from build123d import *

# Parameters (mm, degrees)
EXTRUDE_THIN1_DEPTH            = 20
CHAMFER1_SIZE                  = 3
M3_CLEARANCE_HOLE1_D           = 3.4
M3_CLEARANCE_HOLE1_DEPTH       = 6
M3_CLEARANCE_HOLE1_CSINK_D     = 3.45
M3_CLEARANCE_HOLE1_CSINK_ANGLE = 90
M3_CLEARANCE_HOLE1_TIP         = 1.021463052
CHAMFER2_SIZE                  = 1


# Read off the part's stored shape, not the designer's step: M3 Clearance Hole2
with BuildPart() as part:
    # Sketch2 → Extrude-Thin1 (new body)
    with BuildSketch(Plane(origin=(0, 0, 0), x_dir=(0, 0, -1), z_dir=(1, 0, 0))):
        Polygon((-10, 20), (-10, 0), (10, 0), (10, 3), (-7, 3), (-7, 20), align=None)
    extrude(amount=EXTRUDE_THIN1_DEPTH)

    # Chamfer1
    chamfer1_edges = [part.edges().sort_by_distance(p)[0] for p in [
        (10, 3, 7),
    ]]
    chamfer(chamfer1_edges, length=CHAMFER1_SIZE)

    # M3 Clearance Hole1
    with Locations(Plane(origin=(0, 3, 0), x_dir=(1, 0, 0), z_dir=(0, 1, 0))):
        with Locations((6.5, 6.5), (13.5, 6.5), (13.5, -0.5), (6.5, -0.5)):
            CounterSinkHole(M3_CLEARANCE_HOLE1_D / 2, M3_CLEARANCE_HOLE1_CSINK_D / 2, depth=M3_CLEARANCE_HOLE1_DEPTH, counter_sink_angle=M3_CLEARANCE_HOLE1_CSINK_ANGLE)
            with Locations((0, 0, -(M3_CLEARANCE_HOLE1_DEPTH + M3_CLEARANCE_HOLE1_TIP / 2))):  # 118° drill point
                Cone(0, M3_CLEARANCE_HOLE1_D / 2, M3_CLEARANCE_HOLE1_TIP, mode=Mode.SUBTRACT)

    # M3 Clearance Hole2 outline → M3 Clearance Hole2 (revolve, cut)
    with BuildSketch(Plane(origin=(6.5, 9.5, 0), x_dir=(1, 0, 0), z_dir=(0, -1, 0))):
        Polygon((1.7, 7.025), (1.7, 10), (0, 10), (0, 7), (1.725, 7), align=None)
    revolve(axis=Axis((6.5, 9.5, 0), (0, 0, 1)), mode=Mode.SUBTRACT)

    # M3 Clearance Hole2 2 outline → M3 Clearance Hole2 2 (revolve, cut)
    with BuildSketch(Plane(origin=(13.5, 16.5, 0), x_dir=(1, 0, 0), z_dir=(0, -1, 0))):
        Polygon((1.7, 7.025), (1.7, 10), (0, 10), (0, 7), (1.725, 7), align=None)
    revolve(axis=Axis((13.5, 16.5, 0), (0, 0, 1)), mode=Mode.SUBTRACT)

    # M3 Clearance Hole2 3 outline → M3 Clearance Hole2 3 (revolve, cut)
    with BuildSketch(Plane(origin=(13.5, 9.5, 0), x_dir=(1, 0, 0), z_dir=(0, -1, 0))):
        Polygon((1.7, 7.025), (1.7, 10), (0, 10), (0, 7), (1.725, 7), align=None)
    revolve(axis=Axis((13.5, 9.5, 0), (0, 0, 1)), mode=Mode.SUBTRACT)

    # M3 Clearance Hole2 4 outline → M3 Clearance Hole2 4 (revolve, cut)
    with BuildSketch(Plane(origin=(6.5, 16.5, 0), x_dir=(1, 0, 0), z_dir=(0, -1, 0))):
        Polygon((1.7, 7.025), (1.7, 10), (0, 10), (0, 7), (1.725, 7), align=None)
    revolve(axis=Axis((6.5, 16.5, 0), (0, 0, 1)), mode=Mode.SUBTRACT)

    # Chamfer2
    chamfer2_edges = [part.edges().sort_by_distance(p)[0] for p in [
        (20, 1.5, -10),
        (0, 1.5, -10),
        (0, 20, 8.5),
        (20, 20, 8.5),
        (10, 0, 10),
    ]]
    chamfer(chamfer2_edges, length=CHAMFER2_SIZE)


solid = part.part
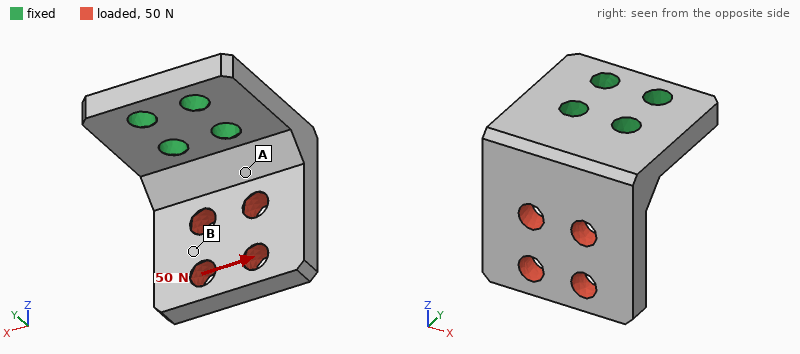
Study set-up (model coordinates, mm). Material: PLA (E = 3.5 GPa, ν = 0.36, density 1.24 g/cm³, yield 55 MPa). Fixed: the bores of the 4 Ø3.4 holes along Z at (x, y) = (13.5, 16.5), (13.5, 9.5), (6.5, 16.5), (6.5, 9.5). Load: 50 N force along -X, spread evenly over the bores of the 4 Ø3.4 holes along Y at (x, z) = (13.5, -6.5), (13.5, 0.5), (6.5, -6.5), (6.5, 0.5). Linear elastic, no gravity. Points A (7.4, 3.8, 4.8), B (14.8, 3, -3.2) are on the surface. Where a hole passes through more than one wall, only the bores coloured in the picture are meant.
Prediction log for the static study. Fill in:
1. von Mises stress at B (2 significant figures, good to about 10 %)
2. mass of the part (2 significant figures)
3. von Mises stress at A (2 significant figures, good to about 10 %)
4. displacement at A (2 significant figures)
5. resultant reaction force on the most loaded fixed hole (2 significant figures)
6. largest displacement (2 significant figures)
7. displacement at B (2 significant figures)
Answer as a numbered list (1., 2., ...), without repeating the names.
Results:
1. 2.0 MPa
2. 2.6 g
3. 7.2 MPa
4. 0.025 mm
5. 65 N
6. 0.13 mm
7. 0.081 mm
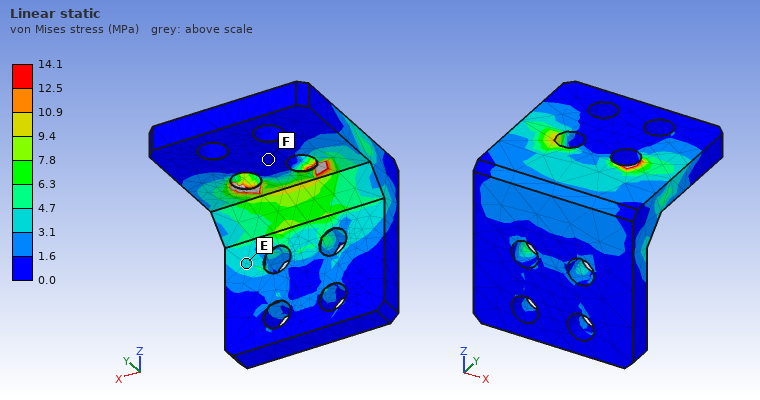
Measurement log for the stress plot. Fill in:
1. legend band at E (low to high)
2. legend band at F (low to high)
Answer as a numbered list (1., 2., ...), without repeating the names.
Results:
1. 3.1 to 4.7 MPa
2. 0.0 to 1.6 MPa
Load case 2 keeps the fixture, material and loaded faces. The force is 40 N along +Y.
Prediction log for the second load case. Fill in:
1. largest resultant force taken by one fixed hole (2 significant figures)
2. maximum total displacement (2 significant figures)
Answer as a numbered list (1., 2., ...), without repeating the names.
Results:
1. 21 N
2. 0.40 mm
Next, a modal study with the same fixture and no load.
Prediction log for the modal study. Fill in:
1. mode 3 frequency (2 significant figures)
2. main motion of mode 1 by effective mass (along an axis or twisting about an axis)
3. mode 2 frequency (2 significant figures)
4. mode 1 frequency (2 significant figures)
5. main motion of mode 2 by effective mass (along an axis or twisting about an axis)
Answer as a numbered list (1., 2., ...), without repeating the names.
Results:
1. 5400 Hz
2. along Y
3. 3500 Hz
4. 2000 Hz
5. along X
